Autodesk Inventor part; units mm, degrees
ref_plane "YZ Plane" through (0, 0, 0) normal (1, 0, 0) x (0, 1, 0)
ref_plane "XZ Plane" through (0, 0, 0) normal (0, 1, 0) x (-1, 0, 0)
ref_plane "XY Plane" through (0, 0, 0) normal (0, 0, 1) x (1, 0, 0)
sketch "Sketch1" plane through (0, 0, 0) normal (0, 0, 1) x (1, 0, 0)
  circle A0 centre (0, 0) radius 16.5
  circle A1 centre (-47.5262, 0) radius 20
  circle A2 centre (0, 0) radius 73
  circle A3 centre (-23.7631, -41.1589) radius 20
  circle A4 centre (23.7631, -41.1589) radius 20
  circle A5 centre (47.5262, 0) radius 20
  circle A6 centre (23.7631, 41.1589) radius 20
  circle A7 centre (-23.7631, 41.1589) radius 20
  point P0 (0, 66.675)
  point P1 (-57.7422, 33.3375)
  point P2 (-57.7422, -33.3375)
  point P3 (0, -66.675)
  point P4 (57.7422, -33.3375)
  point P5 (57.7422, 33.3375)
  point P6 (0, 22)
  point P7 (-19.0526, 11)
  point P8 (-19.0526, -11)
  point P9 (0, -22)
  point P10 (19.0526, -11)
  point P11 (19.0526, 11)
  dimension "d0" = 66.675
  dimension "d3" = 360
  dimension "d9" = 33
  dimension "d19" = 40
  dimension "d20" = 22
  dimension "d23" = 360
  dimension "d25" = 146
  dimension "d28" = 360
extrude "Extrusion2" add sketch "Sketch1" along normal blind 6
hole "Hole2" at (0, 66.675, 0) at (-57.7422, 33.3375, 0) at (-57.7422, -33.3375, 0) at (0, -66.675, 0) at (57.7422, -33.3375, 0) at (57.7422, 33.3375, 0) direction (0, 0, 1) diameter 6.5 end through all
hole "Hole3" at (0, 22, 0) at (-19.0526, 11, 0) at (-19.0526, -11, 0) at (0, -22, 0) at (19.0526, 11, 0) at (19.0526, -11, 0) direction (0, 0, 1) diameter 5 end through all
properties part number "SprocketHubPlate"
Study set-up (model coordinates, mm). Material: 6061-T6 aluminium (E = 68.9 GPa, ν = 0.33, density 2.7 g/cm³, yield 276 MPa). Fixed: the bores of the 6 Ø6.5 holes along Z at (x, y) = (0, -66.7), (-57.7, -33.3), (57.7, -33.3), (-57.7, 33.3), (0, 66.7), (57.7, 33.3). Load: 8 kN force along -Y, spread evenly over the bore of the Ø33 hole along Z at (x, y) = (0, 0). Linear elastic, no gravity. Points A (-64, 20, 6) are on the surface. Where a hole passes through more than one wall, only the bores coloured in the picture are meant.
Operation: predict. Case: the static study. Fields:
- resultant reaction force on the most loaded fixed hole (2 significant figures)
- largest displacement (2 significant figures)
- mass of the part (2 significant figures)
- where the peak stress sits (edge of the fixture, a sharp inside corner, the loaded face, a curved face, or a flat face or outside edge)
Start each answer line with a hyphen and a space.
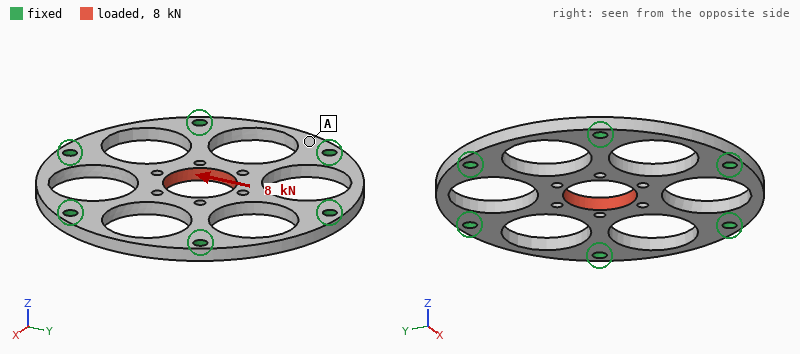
- 2.3 kN
- 26 µm
- 130 g
- a curved face
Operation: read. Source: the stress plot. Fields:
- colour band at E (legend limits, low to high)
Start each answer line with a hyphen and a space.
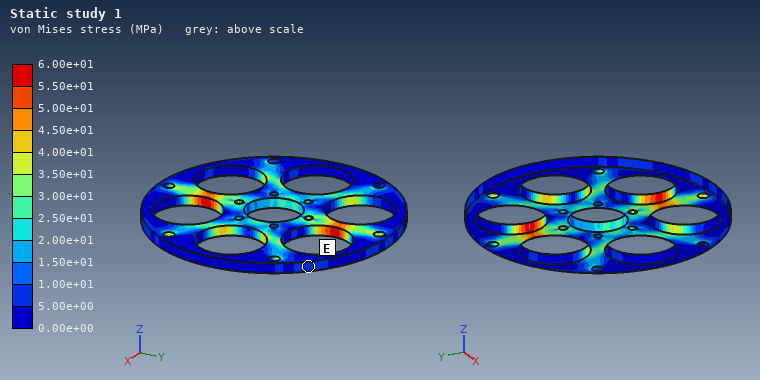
- 5.00e+00 to 1.00e+01 MPa
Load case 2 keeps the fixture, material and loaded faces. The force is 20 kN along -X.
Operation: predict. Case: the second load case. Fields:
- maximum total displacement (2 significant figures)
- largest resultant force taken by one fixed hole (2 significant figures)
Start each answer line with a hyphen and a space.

- 65 µm
- 5.0 kN
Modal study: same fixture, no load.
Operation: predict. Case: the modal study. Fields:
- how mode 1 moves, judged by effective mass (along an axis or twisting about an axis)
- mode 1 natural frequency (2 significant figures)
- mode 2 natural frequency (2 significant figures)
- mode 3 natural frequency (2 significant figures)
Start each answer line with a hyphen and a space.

- along Z
- 2600 Hz
- 5100 Hz
- 5100 Hz
